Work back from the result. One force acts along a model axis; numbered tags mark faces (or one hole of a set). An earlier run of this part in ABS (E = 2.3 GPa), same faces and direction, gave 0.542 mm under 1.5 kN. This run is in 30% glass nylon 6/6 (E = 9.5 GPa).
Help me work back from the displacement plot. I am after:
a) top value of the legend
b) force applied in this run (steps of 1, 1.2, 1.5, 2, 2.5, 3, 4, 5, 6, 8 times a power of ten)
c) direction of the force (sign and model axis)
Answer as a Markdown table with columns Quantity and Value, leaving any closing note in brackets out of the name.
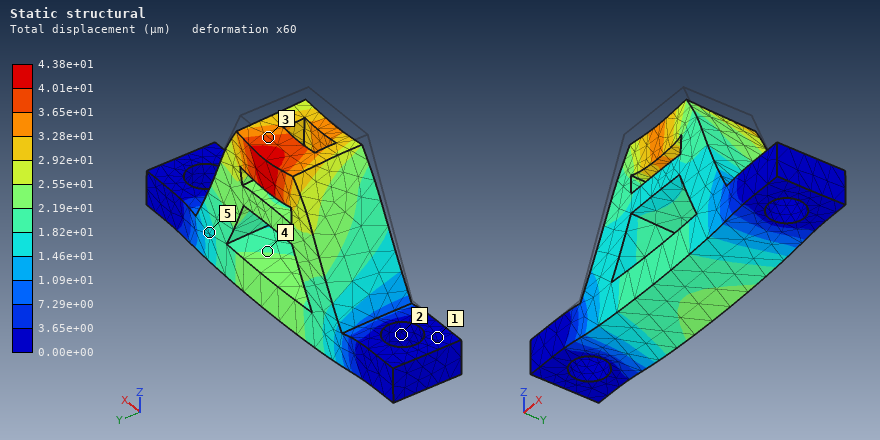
| Quantity | Value |
|---|---|
| top value of the legend | 4.38e+01 µm |
| force applied in this run | 500 N |
| direction of the force | -Z |
